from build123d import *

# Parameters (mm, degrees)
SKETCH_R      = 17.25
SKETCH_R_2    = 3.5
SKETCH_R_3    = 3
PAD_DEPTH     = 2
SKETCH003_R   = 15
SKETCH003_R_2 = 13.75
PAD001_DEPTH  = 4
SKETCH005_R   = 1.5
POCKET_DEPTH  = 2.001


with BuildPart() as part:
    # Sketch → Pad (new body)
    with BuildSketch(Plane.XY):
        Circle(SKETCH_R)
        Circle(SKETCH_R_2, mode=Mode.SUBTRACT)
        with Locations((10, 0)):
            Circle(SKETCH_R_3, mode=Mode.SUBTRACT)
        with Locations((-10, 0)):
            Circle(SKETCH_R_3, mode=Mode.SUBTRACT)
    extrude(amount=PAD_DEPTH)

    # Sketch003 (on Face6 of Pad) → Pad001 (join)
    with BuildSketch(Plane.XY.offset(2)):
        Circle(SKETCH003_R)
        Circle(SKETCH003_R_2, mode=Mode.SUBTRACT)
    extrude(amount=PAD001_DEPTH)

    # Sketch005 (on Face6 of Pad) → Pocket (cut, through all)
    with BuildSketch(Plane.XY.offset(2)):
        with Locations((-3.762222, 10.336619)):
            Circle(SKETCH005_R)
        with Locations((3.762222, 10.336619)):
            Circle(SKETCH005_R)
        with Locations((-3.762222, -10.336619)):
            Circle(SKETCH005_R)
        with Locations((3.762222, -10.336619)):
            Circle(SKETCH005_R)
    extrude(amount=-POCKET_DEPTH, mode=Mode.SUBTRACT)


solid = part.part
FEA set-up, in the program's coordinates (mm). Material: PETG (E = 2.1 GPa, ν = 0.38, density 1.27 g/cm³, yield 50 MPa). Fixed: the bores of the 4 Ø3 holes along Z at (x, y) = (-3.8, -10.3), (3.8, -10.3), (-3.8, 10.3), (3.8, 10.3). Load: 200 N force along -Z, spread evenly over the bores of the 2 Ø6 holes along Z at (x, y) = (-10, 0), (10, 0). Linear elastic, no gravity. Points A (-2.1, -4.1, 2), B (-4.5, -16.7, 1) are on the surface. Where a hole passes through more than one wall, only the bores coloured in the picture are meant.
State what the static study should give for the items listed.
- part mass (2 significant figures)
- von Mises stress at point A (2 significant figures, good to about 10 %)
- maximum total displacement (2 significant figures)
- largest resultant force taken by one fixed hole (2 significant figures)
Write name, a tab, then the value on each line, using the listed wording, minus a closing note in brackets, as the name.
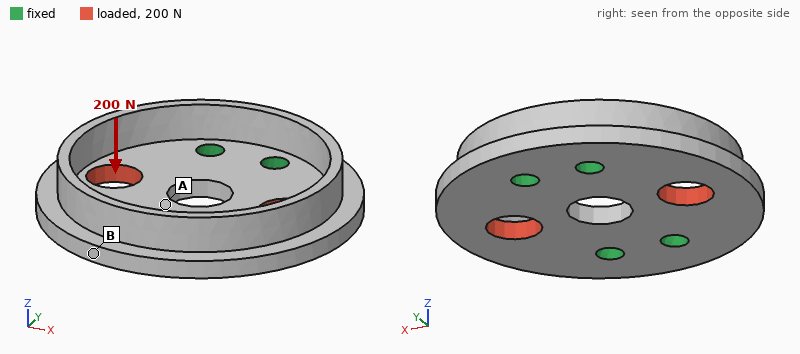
part mass	2.6 g
von Mises stress at point A	13 MPa
maximum total displacement	0.43 mm
largest resultant force taken by one fixed hole	54 N
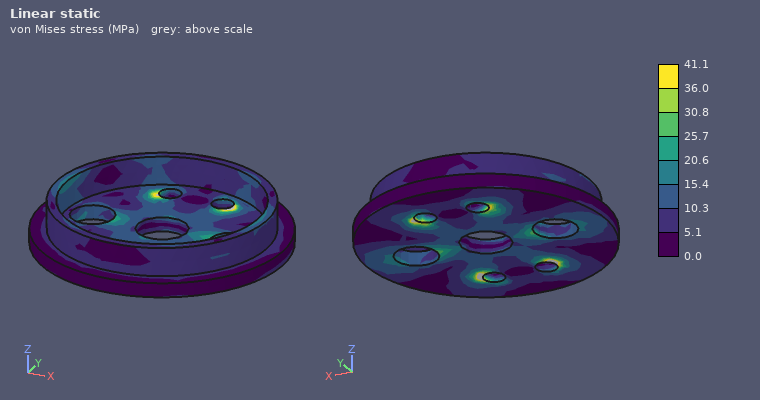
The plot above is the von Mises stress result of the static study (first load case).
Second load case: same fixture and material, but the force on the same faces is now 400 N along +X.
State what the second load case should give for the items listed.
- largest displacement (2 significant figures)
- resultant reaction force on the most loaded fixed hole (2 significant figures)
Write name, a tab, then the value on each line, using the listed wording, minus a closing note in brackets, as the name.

largest displacement	62 µm
resultant reaction force on the most loaded fixed hole	100 N
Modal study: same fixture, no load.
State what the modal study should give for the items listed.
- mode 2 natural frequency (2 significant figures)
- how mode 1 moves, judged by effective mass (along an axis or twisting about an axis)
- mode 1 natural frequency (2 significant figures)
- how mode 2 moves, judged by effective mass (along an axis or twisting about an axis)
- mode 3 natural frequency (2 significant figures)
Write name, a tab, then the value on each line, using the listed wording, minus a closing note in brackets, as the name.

mode 2 natural frequency	3400 Hz
how mode 1 moves, judged by effective mass	along Z
mode 1 natural frequency	3200 Hz
how mode 2 moves, judged by effective mass	twisting about Y
mode 3 natural frequency	6300 Hz
